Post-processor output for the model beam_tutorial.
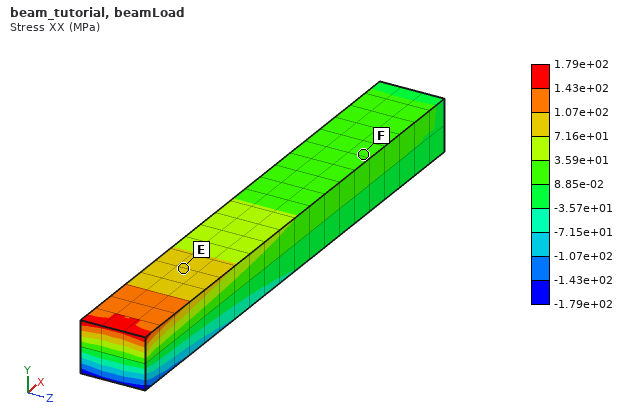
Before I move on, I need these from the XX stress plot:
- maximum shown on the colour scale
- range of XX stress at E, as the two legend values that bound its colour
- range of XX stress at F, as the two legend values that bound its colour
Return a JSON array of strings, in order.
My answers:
["1.79e+02 MPa", "7.16e+01 to 1.07e+02 MPa", "8.85e-02 to 3.59e+01 MPa"]
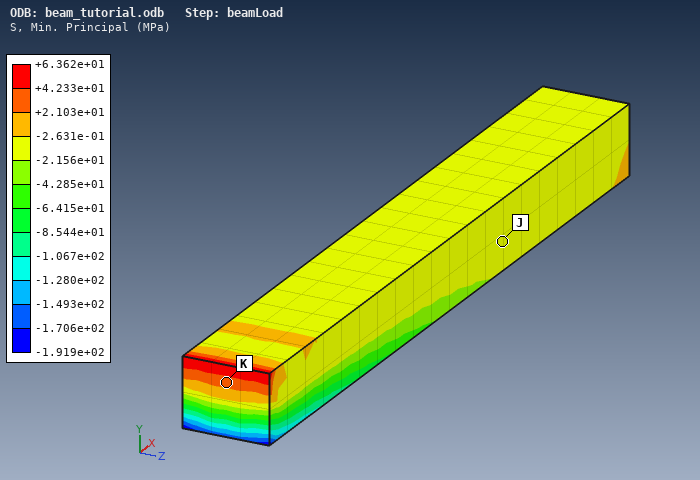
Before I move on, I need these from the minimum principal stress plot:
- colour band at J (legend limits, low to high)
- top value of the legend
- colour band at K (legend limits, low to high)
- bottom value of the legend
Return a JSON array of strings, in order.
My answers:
["-2.156e+01 to -2.631e-01 MPa", "+6.362e+01 MPa", "+2.103e+01 to +4.233e+01 MPa", "-1.919e+02 MPa"]
